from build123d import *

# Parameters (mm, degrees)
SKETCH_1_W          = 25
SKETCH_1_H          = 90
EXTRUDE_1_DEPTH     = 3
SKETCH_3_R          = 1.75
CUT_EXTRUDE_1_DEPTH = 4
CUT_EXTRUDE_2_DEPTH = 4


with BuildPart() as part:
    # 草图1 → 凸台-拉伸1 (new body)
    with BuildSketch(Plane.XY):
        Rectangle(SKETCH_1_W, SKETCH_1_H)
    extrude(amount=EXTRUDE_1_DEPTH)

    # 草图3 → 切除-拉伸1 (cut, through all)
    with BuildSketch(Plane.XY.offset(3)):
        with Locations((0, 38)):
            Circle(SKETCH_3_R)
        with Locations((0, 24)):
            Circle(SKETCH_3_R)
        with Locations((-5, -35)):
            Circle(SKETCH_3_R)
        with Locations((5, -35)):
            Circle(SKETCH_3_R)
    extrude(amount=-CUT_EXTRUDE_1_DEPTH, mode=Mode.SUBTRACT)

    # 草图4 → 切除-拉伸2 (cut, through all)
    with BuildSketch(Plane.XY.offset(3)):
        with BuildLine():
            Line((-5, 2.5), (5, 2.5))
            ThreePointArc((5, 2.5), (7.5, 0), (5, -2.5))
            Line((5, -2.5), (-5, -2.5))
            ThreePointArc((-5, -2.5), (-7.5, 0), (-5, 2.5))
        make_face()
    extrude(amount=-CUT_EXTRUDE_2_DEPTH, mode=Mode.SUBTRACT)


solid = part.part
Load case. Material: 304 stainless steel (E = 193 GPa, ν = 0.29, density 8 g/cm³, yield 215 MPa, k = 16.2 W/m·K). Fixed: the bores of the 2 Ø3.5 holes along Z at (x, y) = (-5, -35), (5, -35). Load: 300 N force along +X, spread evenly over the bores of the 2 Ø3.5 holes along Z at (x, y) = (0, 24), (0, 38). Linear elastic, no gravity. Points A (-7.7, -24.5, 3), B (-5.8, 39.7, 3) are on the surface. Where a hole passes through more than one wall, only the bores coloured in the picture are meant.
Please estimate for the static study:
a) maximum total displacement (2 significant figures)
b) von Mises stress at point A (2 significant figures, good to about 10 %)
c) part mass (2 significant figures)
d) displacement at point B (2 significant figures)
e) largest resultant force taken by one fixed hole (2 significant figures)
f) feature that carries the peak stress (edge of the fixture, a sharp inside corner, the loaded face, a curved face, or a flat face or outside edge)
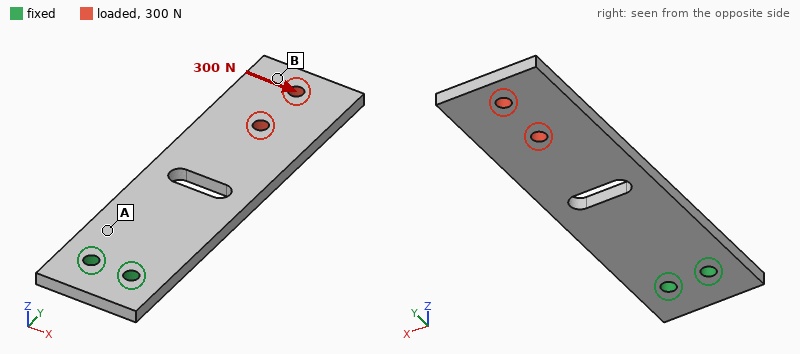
71 µm
35 MPa
51 g
65 µm
1.6 kN
edge of the fixture
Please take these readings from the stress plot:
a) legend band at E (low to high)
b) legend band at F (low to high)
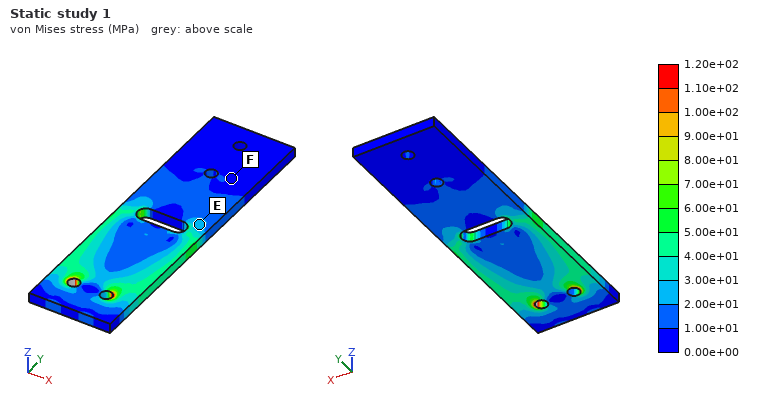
2.00e+01 to 3.00e+01 MPa
0.00e+00 to 1.00e+01 MPa
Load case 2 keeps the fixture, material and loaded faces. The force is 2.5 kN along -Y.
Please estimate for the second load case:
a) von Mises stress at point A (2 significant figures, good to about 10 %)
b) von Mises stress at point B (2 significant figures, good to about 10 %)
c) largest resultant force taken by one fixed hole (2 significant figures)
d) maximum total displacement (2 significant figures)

35 MPa
15 MPa
1.3 kN
17 µm
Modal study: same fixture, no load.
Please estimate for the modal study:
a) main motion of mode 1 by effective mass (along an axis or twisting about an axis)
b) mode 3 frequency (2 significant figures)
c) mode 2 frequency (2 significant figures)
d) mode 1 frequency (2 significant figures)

along Z
2200 Hz
2200 Hz
360 Hz
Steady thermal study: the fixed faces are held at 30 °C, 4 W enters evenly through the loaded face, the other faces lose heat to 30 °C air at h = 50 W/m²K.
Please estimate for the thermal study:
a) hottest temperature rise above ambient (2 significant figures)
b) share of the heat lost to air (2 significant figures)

46 K
96 %
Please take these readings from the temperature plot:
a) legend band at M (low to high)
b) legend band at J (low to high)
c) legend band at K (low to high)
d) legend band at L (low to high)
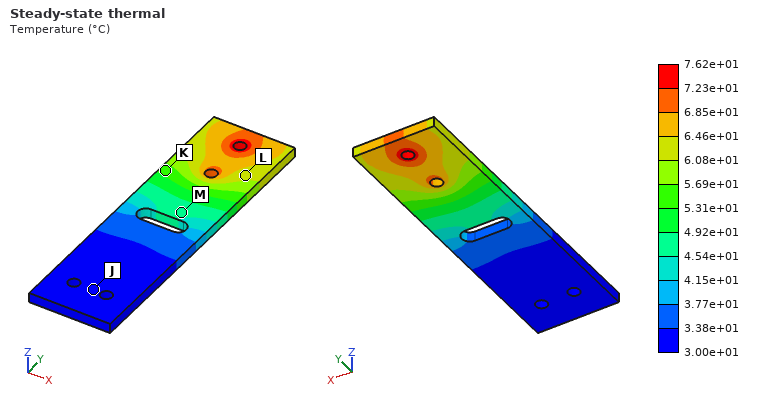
4.54e+01 to 4.92e+01 °C
3.00e+01 to 3.38e+01 °C
5.31e+01 to 5.69e+01 °C
6.08e+01 to 6.46e+01 °C
